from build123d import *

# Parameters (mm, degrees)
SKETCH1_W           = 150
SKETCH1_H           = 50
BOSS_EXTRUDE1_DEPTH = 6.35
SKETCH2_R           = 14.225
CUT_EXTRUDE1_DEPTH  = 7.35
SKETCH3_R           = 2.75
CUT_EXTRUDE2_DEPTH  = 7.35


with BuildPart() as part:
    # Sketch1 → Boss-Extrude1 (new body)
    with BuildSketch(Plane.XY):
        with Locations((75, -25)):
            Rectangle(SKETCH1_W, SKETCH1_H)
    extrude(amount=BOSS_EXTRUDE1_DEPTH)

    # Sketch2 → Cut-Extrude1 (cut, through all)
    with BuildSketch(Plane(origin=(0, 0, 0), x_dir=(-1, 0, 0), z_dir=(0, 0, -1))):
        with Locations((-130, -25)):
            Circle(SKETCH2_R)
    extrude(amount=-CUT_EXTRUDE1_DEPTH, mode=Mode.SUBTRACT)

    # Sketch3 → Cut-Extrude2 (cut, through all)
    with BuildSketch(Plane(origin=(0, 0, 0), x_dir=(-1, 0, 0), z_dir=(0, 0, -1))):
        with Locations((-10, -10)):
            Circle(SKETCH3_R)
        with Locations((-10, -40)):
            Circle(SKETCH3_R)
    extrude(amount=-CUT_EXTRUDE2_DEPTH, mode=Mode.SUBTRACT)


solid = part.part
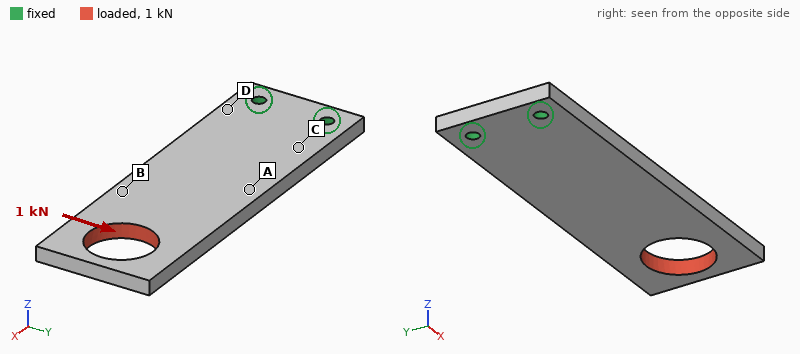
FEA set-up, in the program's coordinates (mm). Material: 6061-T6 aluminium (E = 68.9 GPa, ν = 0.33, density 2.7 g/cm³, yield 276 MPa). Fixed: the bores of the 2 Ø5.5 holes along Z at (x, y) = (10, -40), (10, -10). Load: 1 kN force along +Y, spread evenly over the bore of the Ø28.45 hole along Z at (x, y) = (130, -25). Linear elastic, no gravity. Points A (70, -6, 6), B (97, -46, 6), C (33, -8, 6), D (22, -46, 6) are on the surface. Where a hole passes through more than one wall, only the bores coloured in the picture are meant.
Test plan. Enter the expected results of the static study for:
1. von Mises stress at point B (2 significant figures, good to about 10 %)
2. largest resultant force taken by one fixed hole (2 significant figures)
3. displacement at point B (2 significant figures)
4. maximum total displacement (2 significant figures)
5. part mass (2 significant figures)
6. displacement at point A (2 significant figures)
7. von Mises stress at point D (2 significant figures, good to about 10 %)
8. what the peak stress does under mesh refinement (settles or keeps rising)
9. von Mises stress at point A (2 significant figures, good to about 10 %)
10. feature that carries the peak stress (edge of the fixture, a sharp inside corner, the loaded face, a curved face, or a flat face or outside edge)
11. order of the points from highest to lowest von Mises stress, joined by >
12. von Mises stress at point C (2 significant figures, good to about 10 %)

11 MPa
3.7 kN
0.10 mm
0.21 mm
120 g
0.060 mm
32 MPa
keeps rising
17 MPa
edge of the fixture
D > C > A > B
25 MPa
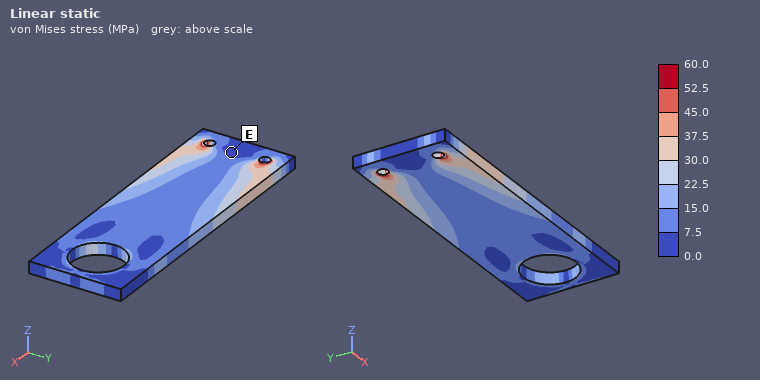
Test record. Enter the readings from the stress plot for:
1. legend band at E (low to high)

0.0 to 7.5 MPa
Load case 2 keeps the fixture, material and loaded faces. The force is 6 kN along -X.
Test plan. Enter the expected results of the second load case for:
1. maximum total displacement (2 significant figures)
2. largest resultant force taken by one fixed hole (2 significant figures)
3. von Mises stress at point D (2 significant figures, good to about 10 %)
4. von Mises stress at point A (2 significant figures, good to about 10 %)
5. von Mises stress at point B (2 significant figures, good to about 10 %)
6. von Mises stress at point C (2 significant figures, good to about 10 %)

67 µm
3.0 kN
19 MPa
19 MPa
24 MPa
19 MPa
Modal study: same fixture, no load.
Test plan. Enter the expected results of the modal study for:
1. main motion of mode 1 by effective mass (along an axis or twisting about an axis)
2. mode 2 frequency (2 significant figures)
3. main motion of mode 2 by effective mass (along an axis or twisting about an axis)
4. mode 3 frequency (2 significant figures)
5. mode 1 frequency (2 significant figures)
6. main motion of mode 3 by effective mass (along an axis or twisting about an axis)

along Z
1500 Hz
twisting about X
1700 Hz
300 Hz
along Z
